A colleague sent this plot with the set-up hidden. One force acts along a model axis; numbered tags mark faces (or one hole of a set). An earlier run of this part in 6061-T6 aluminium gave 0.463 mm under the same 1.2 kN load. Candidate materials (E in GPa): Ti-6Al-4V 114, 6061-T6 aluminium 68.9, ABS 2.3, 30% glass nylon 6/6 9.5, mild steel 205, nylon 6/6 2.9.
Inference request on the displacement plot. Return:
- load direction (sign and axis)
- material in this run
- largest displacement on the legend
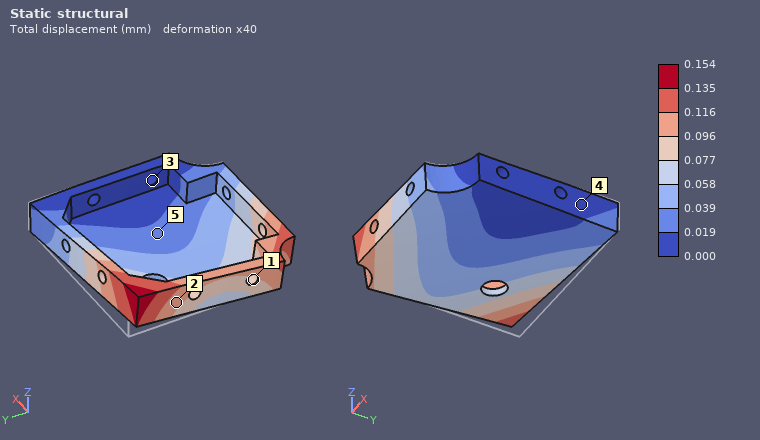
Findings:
-Y
mild steel
0.154 mm
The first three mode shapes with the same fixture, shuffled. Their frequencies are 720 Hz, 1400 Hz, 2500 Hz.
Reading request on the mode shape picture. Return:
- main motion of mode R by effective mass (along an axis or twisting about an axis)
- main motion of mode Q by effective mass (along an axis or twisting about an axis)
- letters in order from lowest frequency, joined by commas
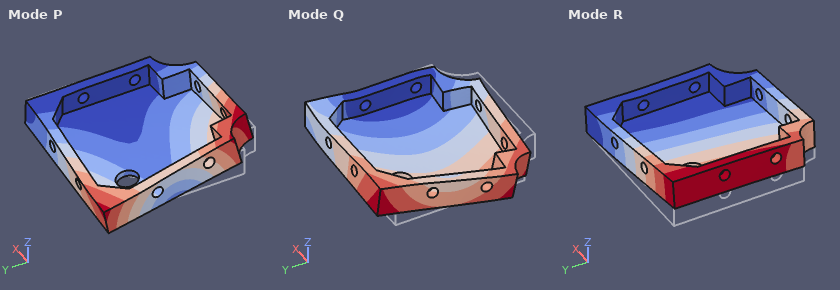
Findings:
along Z
along Y
R, P, Q
